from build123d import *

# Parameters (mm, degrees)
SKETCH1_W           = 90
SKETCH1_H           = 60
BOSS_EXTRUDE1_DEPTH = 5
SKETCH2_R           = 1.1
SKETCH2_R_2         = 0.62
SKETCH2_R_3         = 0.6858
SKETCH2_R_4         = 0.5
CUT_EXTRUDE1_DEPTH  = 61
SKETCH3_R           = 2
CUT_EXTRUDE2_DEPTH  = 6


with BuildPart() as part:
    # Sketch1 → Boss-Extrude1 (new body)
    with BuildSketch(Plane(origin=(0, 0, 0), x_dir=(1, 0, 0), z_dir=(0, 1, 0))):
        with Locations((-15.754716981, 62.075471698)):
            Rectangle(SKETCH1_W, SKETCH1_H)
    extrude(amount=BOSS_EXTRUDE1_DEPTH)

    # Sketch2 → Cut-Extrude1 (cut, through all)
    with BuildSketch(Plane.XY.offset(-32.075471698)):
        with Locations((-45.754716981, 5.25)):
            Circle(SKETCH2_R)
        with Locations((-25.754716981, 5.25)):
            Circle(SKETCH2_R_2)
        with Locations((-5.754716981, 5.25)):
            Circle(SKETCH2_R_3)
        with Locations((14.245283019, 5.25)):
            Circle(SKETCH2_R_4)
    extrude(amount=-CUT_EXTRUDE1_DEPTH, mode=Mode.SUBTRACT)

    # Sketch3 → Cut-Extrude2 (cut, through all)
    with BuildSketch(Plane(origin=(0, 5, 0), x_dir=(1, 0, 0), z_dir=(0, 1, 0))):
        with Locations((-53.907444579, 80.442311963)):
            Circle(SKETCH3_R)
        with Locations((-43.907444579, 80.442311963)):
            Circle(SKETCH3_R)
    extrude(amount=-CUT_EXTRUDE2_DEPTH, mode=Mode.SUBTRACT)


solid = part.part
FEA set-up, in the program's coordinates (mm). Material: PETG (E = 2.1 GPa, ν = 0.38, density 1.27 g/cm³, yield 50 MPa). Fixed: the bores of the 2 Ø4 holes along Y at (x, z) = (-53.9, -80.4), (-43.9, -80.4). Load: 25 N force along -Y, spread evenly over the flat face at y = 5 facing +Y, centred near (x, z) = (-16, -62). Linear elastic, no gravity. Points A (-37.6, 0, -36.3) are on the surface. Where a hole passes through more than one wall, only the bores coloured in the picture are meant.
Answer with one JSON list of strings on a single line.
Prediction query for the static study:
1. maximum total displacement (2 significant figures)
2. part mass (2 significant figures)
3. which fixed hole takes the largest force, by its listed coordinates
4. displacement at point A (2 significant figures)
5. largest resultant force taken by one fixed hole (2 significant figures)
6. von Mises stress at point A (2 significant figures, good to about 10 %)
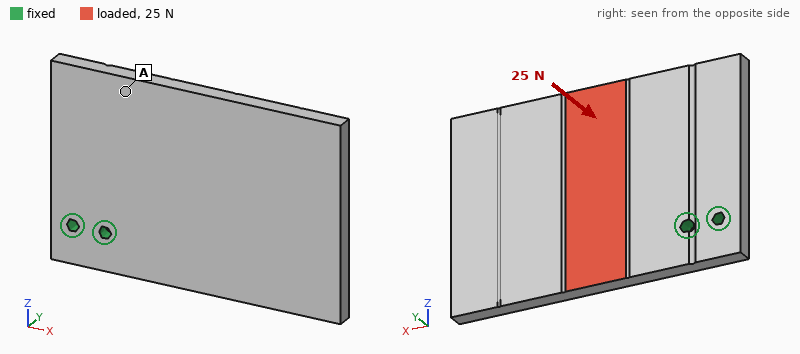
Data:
["1.2 mm", "34 g", "(-43.9, -80.4)", "0.35 mm", "52 N", "0.82 MPa"]
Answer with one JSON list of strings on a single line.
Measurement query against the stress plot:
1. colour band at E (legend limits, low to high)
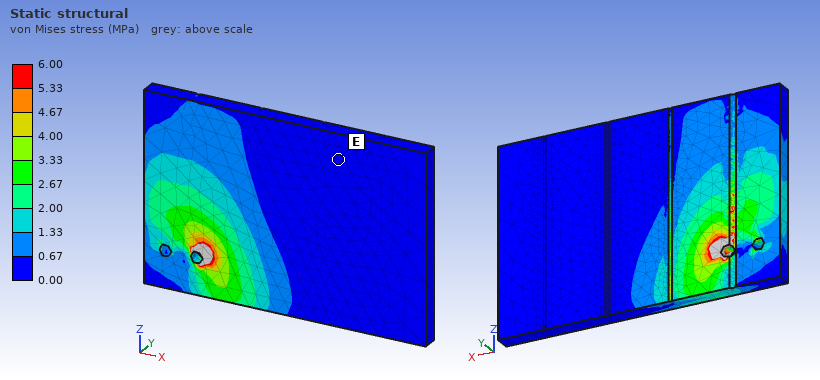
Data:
["0.00 to 0.67 MPa"]
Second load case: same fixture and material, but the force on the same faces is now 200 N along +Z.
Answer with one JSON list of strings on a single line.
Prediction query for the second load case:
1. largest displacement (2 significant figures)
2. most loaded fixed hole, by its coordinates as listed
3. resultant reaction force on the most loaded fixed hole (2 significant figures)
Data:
["0.93 mm", "(-43.9, -80.4)", "580 N"]
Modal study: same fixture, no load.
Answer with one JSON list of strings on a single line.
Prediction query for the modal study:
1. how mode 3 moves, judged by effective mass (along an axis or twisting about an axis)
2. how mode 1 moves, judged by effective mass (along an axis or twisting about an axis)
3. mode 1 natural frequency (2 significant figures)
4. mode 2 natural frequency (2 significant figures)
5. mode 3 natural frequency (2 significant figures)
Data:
["along Z", "along Y", "150 Hz", "320 Hz", "520 Hz"]
